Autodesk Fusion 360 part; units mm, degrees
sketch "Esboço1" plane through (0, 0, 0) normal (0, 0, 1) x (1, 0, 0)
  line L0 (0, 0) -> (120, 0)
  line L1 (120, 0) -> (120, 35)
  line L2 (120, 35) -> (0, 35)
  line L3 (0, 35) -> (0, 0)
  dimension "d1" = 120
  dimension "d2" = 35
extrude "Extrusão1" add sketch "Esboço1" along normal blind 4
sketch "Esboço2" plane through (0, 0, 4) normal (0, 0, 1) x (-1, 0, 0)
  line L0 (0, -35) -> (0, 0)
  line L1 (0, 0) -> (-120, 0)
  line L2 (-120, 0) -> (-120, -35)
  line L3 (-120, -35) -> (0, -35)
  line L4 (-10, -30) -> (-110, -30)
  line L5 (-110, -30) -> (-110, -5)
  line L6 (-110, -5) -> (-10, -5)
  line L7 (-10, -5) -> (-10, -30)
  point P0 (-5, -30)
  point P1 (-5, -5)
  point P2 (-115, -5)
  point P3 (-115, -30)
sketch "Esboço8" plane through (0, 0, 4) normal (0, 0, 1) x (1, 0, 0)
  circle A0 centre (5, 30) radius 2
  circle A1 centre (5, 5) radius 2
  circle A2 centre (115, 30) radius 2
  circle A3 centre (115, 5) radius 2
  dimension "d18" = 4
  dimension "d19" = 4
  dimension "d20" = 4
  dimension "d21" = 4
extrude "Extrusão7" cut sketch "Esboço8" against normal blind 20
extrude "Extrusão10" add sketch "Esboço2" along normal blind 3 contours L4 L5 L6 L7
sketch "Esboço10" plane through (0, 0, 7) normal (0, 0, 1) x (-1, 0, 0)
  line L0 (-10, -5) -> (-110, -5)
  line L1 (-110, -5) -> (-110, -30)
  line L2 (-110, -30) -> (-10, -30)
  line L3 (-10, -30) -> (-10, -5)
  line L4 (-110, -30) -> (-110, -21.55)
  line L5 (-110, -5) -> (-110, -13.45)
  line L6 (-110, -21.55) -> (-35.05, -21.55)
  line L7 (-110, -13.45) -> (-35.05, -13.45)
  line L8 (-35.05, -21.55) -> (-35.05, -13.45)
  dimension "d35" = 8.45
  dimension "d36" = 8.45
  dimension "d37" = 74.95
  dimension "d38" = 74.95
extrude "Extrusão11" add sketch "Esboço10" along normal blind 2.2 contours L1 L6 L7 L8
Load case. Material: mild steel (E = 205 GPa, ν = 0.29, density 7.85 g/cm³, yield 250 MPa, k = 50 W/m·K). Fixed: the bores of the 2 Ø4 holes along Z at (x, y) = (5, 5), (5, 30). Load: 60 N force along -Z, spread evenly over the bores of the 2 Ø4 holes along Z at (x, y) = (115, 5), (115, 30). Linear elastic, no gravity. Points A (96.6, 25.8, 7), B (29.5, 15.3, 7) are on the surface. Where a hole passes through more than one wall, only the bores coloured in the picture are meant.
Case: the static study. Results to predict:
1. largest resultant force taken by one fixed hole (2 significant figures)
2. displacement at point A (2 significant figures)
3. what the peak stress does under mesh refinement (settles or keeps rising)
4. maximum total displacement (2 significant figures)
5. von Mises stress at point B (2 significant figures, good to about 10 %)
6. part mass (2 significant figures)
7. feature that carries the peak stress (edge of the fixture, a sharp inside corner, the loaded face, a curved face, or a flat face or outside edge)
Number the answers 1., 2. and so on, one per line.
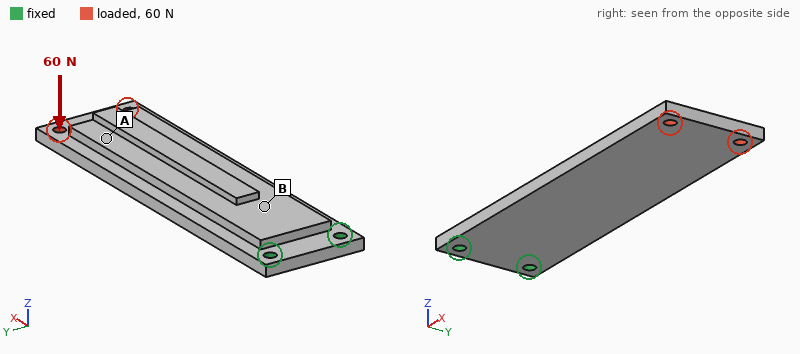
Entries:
1. 38 N
2. 0.19 mm
3. keeps rising
4. 0.26 mm
5. 25 MPa
6. 200 g
7. edge of the fixture
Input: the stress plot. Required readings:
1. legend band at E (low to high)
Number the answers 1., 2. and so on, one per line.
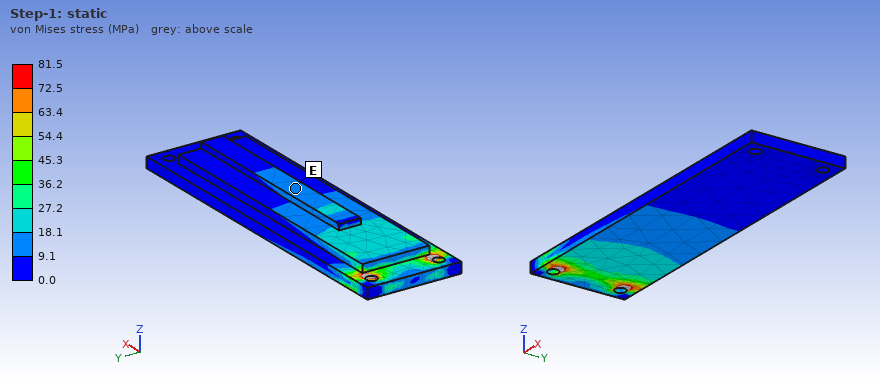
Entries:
1. 9.1 to 18.1 MPa
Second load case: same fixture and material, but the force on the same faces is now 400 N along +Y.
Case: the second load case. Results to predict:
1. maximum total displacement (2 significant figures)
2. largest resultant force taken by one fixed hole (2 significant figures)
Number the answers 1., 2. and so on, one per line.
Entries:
1. 61 µm
2. 1.7 kN
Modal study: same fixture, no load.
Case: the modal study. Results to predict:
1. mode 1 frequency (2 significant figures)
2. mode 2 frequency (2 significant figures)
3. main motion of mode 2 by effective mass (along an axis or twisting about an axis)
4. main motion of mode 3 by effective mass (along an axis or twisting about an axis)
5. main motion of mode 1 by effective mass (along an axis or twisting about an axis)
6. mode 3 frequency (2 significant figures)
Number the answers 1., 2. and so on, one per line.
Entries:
1. 330 Hz
2. 1900 Hz
3. along Y
4. along Z
5. along Z
6. 2600 Hz
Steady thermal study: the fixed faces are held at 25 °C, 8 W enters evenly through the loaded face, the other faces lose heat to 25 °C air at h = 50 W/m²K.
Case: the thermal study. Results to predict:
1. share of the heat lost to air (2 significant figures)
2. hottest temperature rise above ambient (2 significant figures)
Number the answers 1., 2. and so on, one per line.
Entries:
1. 82 %
2. 39 K
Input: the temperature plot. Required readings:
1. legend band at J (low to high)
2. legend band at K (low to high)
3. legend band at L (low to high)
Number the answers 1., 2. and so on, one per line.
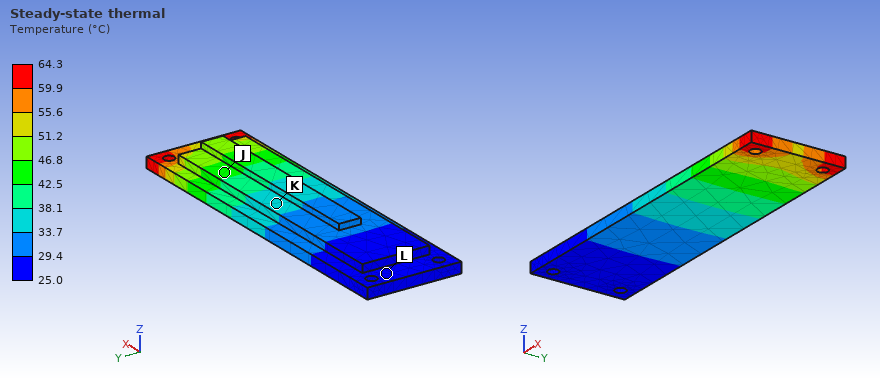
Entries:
1. 42.5 to 46.8 °C
2. 33.7 to 38.1 °C
3. 25.0 to 29.4 °C
